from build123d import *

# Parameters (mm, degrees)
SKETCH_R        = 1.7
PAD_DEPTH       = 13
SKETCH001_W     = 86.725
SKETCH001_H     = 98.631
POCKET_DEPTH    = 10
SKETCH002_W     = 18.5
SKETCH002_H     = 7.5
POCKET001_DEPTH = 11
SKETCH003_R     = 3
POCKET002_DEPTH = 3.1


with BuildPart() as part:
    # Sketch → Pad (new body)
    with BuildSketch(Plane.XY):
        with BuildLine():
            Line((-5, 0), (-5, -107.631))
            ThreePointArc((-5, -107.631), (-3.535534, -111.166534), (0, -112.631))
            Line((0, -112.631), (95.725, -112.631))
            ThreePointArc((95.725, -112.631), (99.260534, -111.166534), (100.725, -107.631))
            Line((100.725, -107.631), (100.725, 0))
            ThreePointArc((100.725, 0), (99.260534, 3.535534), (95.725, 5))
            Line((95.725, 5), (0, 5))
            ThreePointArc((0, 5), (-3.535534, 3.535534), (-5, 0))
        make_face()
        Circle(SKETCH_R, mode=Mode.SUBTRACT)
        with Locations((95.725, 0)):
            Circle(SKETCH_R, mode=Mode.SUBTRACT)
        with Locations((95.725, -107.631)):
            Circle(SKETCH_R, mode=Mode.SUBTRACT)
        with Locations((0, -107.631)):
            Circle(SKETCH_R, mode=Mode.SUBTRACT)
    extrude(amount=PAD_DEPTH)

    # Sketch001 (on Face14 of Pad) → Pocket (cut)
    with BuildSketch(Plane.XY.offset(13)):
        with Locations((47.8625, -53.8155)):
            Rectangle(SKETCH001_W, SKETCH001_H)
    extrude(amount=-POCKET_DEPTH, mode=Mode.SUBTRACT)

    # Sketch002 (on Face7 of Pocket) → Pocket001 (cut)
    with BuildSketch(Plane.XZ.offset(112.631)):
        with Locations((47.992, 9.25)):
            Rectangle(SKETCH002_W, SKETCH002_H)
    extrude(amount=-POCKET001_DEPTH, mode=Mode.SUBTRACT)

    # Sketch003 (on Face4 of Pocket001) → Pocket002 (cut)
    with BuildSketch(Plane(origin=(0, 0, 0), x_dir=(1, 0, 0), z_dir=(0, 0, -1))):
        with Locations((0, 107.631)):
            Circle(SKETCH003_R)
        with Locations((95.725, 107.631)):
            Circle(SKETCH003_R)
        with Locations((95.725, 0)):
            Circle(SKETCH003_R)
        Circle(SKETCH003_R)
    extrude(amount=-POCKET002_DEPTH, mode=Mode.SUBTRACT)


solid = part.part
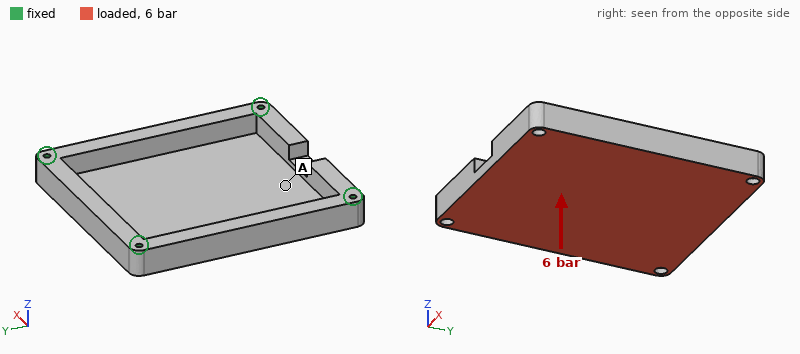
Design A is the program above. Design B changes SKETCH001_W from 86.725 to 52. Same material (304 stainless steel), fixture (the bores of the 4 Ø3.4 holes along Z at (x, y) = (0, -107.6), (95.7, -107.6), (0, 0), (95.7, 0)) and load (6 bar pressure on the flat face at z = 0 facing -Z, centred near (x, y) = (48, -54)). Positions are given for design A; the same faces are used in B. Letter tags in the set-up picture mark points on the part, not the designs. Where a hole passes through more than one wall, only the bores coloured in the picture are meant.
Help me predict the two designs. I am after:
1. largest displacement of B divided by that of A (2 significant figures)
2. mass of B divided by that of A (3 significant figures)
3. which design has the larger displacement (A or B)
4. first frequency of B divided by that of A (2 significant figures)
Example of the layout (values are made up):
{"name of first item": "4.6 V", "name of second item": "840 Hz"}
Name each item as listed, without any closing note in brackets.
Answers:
{"largest displacement of B divided by that of A": "0.35", "mass of B divided by that of A": "1.46", "which design has the larger displacement": "A", "first frequency of B divided by that of A": "1.4"}
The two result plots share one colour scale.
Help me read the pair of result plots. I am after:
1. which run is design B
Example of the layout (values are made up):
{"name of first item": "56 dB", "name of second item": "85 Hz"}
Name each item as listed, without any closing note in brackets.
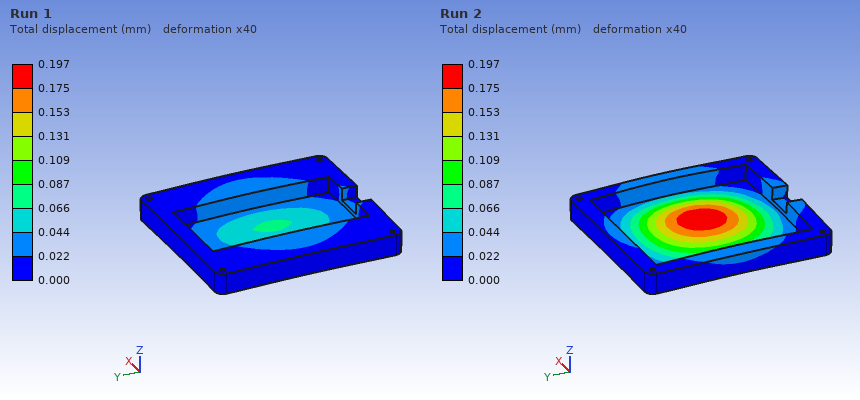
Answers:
{"which run is design B": "Run 1"}
